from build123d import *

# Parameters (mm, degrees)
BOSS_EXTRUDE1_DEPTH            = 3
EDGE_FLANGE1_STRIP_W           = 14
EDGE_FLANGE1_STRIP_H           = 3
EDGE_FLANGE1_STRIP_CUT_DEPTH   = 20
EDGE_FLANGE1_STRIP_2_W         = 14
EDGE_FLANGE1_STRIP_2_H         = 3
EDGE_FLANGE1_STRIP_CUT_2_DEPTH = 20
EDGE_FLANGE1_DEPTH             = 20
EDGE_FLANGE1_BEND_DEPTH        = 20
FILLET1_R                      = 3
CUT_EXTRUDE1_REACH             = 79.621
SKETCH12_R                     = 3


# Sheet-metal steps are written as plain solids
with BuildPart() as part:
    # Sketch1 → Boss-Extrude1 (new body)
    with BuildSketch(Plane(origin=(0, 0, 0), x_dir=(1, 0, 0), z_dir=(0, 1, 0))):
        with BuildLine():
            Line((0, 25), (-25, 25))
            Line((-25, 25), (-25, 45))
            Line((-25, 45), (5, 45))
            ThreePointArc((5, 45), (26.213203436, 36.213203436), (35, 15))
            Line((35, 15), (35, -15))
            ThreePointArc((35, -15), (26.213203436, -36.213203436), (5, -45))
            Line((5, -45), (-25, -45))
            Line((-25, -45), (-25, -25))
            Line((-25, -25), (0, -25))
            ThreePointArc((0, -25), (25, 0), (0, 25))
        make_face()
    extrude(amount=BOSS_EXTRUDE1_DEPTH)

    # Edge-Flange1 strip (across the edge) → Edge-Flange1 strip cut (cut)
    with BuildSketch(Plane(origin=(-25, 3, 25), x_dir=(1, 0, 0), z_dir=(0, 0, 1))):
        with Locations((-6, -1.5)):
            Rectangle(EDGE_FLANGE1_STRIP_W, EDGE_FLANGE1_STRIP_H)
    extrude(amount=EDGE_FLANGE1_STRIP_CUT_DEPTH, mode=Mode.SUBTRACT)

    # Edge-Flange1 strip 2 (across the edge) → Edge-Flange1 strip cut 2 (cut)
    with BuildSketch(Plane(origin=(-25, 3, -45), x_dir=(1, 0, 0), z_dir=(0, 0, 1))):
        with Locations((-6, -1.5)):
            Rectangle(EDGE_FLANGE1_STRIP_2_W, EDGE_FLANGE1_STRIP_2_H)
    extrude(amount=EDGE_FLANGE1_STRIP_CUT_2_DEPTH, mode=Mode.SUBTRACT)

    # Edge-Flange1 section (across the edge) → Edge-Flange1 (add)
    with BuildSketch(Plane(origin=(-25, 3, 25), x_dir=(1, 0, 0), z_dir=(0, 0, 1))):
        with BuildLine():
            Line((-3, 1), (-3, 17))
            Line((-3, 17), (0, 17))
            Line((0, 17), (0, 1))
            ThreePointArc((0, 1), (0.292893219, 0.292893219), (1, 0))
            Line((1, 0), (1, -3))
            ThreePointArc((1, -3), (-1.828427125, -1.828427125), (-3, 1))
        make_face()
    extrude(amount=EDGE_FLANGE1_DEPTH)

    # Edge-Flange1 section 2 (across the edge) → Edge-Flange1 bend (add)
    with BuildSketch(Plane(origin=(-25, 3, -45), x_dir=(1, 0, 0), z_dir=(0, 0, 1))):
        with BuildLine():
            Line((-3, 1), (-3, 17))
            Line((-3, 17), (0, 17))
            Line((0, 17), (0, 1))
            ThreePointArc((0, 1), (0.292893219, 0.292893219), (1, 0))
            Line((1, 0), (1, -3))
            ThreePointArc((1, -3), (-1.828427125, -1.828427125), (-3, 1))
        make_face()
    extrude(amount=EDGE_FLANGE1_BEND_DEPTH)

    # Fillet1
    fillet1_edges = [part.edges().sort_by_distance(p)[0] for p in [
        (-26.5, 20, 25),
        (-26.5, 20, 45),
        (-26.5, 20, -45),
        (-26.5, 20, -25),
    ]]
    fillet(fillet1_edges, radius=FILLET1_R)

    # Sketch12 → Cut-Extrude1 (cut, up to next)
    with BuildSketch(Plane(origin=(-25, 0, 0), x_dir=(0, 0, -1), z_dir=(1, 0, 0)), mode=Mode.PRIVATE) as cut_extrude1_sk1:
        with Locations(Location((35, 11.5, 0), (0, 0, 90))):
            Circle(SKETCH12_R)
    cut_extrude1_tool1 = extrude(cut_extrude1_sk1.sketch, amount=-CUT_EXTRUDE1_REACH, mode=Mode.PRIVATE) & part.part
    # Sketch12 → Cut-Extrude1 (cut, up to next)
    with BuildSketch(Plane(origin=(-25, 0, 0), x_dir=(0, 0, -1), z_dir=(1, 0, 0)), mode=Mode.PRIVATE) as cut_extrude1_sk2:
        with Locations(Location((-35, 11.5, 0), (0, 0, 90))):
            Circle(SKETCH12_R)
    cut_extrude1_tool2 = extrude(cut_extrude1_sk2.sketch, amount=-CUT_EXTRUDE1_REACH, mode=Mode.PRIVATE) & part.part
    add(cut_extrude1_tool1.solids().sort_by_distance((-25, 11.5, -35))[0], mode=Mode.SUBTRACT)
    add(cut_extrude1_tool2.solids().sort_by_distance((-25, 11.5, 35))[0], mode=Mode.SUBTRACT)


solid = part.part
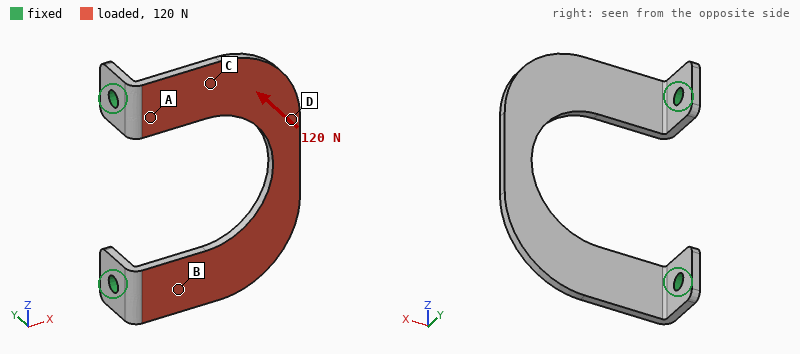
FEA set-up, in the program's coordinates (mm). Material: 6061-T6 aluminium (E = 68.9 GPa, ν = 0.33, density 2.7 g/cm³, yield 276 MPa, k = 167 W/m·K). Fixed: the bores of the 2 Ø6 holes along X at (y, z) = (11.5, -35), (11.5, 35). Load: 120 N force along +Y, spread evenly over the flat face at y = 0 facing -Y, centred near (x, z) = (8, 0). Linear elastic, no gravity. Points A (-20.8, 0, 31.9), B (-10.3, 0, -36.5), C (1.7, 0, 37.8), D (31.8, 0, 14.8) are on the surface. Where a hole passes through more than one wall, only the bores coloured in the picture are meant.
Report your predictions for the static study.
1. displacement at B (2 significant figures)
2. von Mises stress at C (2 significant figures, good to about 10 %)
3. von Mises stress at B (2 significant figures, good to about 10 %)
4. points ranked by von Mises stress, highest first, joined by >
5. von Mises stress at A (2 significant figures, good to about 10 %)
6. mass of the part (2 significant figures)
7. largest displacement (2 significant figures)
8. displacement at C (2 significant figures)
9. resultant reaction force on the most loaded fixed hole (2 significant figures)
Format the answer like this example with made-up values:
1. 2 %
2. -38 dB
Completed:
1. 0.16 mm
2. 23 MPa
3. 38 MPa
4. A > B > C > D
5. 53 MPa
6. 28 g
7. 0.98 mm
8. 0.33 mm
9. 60 N
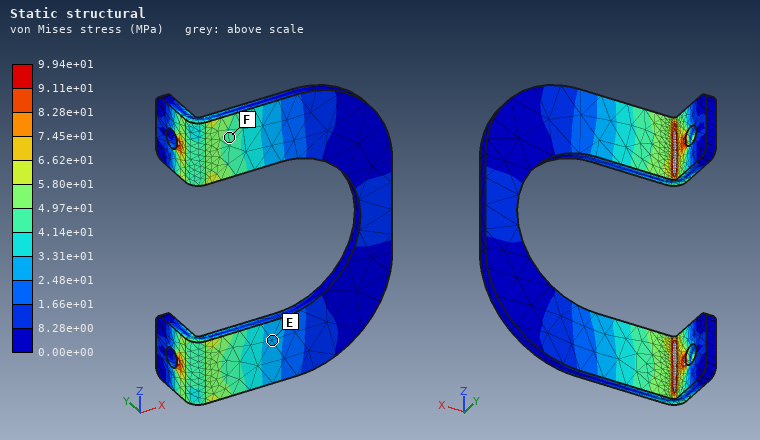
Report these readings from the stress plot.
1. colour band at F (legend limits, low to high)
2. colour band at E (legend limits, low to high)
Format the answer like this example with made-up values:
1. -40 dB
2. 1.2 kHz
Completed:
1. 4.14e+01 to 4.97e+01 MPa
2. 2.48e+01 to 3.31e+01 MPa
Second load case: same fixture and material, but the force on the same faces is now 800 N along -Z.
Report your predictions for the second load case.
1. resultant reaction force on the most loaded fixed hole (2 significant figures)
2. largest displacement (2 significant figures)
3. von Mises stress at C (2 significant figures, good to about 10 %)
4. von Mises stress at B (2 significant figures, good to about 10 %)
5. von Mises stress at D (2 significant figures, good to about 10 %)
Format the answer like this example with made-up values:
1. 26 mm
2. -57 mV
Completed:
1. 510 N
2. 0.16 mm
3. 14 MPa
4. 17 MPa
5. 27 MPa
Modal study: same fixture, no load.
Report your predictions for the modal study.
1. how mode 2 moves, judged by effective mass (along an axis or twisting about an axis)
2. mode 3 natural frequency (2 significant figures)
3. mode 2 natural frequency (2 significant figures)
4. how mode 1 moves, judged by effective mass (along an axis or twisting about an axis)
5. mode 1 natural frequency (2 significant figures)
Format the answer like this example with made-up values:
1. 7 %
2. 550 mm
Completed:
1. twisting about X
2. 2500 Hz
3. 1100 Hz
4. along Y
5. 460 Hz
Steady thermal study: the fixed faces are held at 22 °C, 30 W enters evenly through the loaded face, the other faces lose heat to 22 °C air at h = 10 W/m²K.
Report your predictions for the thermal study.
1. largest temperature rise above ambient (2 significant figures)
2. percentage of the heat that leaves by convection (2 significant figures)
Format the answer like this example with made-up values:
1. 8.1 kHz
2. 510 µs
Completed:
1. 64 K
2. 6.1 %
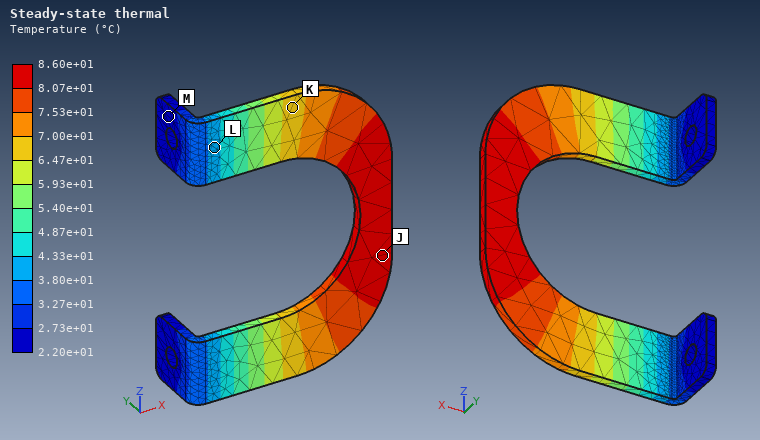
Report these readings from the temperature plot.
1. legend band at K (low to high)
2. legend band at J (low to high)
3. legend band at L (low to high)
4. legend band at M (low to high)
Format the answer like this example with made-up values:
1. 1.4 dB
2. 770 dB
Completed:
1. 6.47e+01 to 7.00e+01 °C
2. 8.07e+01 to 8.60e+01 °C
3. 3.80e+01 to 4.33e+01 °C
4. 2.20e+01 to 2.73e+01 °C
